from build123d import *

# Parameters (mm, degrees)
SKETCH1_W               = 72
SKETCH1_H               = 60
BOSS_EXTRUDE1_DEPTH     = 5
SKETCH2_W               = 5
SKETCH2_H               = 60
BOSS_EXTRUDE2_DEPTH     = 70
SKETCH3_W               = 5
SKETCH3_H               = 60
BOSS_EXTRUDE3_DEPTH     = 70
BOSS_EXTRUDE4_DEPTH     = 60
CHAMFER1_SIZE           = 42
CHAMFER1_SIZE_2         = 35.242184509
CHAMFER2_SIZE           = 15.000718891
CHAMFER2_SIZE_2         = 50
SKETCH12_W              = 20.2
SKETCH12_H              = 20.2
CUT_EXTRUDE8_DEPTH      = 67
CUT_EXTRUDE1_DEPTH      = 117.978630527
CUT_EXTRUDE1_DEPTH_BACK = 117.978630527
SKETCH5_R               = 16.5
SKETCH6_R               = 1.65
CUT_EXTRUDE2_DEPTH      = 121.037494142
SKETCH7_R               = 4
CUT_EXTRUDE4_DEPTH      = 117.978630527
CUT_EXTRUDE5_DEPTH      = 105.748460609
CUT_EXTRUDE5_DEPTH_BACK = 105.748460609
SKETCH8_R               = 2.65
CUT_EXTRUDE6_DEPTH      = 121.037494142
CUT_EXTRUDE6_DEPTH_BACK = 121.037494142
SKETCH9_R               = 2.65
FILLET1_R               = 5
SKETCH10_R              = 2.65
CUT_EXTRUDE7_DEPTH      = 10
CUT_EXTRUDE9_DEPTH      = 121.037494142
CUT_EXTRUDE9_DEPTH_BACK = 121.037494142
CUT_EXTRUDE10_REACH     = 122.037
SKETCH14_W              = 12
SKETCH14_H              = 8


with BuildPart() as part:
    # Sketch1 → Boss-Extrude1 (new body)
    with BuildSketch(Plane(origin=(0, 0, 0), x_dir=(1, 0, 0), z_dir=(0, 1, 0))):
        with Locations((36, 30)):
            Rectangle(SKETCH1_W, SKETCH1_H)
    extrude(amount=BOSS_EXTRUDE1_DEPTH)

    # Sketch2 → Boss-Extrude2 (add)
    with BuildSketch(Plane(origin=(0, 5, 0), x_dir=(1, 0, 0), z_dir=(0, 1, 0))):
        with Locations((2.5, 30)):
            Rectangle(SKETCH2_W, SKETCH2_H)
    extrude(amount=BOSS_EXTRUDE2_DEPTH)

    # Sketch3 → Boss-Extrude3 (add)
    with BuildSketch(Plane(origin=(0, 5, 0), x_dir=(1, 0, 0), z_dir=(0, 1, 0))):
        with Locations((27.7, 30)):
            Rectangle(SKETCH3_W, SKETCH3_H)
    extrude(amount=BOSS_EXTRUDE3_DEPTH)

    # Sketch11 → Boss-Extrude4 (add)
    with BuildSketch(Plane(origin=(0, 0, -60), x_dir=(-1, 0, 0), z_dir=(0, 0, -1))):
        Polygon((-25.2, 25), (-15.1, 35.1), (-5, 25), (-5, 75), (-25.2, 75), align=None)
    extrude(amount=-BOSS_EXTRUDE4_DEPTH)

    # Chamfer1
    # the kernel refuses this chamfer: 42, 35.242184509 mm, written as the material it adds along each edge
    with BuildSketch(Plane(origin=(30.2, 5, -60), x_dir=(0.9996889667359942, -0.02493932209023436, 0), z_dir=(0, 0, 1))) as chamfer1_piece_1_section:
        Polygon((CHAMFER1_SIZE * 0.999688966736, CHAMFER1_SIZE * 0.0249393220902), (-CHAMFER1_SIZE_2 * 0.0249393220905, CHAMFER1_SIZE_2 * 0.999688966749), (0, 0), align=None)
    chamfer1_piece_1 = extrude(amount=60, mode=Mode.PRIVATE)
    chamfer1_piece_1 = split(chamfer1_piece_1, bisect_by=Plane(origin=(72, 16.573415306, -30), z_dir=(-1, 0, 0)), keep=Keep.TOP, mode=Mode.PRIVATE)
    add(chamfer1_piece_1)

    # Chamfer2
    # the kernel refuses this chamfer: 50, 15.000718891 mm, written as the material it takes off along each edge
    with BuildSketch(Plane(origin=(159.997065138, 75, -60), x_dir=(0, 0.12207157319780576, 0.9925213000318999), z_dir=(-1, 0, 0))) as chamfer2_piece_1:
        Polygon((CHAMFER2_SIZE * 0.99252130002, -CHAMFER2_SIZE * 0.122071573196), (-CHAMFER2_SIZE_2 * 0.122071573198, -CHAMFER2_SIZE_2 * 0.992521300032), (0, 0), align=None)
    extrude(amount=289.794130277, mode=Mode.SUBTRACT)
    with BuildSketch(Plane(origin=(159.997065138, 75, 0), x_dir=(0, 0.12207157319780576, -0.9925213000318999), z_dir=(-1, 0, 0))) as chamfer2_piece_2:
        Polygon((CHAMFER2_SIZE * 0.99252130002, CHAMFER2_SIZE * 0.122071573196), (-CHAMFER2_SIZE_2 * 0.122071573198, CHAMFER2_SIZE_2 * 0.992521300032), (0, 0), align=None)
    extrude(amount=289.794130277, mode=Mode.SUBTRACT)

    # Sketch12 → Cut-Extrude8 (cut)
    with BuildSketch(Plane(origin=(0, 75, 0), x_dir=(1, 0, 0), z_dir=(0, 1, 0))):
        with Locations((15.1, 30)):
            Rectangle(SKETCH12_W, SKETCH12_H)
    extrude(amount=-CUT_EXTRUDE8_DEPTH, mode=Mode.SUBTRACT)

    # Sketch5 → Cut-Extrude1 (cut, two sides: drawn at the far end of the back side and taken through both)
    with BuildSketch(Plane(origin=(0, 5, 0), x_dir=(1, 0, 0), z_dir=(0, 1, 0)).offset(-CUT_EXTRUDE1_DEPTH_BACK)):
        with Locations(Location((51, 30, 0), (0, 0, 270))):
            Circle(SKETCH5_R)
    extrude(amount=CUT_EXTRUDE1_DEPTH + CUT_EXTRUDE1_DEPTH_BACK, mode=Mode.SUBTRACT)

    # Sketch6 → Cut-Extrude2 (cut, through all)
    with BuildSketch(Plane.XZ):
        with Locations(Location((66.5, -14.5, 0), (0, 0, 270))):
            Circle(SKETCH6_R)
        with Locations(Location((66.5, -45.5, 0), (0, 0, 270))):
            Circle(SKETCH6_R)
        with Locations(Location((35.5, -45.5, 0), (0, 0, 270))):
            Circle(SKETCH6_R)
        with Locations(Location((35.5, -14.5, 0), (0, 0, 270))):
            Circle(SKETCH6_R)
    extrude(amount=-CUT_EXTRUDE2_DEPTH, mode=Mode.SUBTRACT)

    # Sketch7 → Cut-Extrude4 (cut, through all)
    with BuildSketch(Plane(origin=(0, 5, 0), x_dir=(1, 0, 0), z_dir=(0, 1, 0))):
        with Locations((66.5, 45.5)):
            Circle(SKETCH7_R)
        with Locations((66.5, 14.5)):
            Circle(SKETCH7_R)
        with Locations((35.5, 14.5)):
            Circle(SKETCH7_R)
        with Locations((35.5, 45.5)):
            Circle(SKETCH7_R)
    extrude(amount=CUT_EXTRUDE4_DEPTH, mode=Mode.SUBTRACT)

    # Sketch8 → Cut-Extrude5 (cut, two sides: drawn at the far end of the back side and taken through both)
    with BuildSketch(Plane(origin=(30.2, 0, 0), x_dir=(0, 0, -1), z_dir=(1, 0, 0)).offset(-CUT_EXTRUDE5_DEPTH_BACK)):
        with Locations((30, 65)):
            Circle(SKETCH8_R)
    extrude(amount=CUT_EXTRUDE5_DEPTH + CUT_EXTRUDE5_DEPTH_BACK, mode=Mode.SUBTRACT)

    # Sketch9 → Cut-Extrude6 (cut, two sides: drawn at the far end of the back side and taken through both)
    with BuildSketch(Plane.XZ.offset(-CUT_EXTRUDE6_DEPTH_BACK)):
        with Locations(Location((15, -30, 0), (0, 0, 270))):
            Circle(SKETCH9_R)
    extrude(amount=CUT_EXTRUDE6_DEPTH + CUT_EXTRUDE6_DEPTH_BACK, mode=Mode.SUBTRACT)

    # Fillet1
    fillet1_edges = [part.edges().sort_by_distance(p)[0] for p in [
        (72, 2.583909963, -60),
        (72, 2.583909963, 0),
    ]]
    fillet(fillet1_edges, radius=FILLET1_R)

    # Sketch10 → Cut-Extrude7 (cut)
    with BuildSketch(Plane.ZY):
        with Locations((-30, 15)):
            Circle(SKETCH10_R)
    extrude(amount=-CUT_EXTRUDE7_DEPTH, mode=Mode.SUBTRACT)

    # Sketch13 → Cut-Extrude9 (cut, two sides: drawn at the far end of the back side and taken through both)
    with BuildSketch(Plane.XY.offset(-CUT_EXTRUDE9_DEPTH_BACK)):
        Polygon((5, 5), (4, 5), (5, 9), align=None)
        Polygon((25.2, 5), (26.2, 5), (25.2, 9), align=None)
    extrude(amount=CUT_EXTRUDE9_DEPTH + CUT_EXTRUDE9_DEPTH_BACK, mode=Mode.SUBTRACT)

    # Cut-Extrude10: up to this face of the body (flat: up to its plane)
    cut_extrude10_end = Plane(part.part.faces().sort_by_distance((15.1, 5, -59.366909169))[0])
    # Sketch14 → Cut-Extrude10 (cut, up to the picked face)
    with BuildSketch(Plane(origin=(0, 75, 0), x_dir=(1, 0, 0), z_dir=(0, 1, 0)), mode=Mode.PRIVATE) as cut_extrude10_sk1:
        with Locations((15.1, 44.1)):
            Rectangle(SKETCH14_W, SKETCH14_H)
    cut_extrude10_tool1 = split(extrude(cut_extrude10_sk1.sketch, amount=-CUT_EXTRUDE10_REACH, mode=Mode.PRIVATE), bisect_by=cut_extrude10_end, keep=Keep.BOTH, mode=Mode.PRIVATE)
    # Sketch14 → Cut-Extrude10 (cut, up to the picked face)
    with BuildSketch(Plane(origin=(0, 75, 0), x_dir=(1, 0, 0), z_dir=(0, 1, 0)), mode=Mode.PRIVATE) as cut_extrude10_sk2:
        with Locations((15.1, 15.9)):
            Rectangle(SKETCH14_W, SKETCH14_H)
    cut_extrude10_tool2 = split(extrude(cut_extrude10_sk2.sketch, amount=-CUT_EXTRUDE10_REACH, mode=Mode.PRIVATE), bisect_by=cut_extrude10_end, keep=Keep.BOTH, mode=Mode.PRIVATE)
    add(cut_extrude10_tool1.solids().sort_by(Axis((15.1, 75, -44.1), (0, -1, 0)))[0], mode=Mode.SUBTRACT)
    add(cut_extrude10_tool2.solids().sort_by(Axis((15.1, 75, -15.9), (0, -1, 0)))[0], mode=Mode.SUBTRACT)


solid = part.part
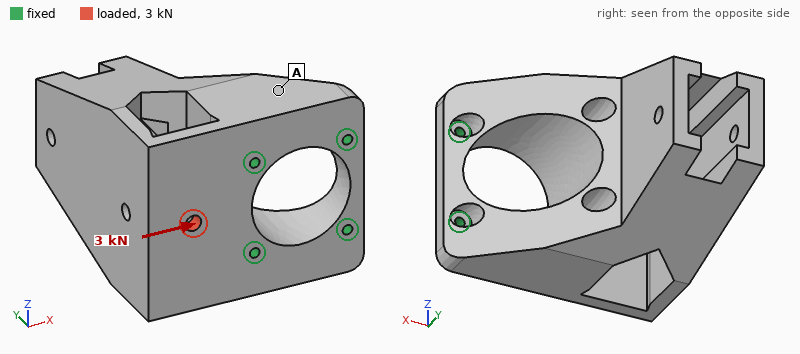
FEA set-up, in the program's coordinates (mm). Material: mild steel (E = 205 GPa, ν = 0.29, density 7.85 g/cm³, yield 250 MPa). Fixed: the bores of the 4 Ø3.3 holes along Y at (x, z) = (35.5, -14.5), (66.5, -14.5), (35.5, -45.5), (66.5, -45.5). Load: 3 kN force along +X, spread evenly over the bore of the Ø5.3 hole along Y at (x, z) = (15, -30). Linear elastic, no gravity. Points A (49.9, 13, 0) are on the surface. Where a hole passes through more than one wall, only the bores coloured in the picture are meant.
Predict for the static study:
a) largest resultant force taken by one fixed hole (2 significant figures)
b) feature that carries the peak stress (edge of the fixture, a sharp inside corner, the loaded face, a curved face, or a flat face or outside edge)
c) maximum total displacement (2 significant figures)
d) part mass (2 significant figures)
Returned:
1.5 kN
the loaded face
3.4 µm
700 g
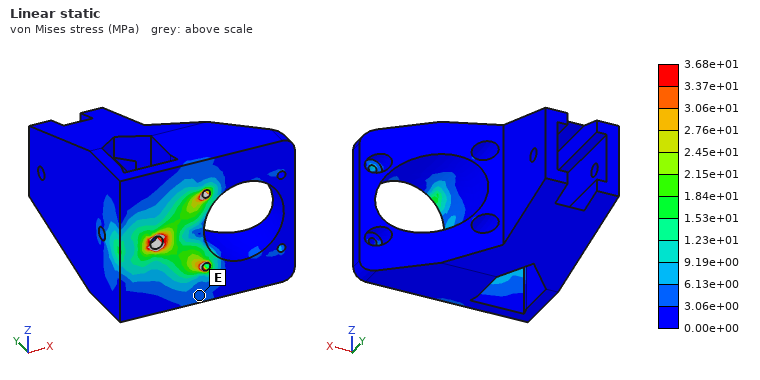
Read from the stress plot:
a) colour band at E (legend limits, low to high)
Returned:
3.06e+00 to 6.13e+00 MPa
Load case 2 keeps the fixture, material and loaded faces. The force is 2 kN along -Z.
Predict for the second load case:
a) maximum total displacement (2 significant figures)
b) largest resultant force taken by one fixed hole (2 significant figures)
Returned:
3.6 µm
1.3 kN
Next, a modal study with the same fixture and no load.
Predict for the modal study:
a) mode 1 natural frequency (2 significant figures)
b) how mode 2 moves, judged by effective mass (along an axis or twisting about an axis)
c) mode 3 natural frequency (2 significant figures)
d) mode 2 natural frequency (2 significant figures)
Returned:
2300 Hz
along Z
7300 Hz
3300 Hz
